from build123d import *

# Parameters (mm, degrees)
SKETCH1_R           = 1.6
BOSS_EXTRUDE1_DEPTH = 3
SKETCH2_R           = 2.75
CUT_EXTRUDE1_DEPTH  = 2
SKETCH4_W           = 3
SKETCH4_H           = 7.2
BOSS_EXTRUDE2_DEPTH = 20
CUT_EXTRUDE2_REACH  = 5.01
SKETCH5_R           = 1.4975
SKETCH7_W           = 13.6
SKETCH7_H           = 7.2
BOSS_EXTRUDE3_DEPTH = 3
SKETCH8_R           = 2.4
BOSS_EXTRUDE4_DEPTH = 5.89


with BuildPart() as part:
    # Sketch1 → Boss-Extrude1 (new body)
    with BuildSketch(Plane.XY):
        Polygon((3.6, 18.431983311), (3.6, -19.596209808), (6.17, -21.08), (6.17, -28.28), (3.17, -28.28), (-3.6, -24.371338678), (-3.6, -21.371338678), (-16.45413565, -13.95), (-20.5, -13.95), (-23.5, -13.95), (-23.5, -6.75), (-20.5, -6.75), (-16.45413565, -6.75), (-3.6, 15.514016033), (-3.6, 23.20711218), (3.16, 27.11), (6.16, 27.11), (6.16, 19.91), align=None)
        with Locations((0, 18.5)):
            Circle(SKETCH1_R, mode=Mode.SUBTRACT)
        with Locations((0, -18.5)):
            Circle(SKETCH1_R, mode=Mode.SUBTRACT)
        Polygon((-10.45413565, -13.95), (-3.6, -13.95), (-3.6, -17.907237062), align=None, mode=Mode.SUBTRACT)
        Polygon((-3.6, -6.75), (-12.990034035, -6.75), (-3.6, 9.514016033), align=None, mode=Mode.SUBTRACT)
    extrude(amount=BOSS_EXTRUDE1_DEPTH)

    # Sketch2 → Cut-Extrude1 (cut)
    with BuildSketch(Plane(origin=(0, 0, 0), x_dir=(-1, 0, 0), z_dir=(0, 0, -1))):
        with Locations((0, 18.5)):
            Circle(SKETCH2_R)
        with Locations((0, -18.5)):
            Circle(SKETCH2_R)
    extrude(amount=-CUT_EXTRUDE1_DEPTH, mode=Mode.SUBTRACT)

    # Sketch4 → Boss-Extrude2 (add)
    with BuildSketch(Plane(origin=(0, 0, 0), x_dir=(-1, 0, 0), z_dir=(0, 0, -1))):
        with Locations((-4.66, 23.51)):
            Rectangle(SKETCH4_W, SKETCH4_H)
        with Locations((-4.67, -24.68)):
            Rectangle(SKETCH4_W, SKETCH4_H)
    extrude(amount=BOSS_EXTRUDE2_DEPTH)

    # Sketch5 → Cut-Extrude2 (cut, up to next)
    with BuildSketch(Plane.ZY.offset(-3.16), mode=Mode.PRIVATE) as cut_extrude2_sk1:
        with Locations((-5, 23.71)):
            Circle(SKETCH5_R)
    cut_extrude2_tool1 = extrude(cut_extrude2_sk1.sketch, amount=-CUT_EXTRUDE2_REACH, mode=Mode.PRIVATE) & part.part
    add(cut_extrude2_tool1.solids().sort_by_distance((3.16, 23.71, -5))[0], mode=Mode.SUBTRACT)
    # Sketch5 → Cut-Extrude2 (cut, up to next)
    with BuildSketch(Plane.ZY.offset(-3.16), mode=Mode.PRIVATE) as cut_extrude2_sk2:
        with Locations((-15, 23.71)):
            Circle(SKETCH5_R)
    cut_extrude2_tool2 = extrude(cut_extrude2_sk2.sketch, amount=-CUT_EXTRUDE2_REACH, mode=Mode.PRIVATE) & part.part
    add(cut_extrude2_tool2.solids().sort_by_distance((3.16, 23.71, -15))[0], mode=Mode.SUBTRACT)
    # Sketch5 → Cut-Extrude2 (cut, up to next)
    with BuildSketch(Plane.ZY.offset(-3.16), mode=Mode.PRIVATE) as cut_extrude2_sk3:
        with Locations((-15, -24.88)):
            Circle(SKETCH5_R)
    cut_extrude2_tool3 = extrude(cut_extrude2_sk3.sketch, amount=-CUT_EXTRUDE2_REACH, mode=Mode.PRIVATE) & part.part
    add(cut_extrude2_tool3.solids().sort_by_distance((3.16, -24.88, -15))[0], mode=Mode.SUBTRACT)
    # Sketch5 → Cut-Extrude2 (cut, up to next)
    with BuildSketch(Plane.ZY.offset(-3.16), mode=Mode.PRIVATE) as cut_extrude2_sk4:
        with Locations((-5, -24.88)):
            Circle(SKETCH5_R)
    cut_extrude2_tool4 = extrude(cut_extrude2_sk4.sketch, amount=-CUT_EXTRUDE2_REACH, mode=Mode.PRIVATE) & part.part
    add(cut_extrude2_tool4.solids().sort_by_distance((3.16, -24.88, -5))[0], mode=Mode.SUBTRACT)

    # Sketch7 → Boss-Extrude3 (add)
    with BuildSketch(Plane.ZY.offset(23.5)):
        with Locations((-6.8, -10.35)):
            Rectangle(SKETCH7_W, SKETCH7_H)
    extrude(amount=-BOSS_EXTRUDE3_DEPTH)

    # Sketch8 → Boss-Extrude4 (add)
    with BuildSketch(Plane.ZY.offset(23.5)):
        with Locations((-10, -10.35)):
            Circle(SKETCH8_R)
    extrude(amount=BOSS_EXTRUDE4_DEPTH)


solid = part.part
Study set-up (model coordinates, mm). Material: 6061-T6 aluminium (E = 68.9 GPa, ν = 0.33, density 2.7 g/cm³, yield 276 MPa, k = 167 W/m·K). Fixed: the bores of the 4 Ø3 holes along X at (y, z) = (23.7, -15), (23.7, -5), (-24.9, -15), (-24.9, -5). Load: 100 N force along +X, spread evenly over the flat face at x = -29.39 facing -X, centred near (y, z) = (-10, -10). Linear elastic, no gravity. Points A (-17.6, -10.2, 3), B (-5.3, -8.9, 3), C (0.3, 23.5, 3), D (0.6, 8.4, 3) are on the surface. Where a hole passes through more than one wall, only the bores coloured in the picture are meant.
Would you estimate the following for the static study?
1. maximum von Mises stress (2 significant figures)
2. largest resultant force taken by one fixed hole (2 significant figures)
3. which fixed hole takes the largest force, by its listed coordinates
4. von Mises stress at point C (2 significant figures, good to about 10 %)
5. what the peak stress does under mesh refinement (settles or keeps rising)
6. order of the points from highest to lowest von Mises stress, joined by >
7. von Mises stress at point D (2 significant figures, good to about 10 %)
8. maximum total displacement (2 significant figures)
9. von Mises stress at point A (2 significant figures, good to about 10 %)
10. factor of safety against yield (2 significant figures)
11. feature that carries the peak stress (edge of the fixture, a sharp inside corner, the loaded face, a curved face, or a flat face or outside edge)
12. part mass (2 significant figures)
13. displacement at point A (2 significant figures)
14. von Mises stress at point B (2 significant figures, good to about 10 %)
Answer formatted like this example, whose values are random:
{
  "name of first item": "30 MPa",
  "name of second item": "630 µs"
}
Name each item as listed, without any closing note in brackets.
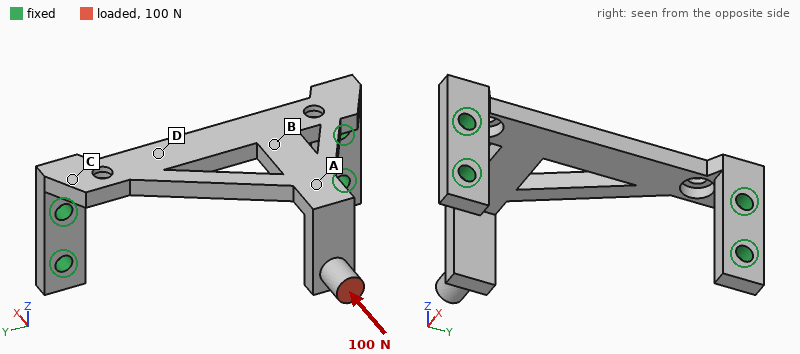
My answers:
{
  "maximum von Mises stress": "210 MPa",
  "largest resultant force taken by one fixed hole": "76 N",
  "which fixed hole takes the largest force, by its listed coordinates": "(-24.9, -5)",
  "von Mises stress at point C": "39 MPa",
  "what the peak stress does under mesh refinement": "settles",
  "order of the points from highest to lowest von Mises stress, joined by >": "A > B > C > D",
  "von Mises stress at point D": "24 MPa",
  "maximum total displacement": "0.75 mm",
  "von Mises stress at point A": "96 MPa",
  "factor of safety against yield": "1.3",
  "feature that carries the peak stress": "a curved face",
  "part mass": "8.2 g",
  "displacement at point A": "0.29 mm",
  "von Mises stress at point B": "54 MPa"
}
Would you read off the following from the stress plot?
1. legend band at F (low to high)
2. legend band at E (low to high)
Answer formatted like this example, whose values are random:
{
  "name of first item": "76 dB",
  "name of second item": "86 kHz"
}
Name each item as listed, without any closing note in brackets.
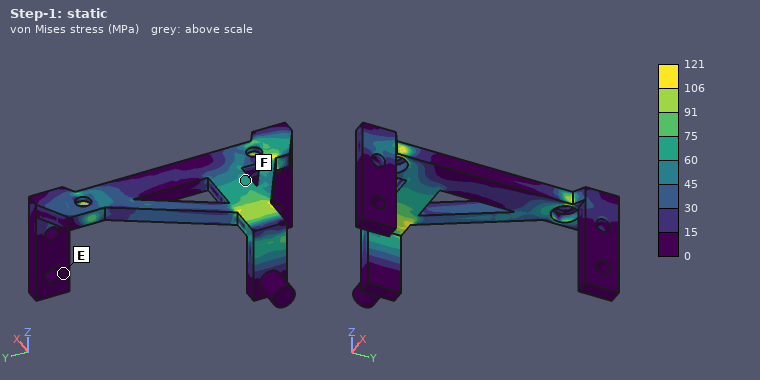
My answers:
{
  "legend band at F": "60 to 75 MPa",
  "legend band at E": "0 to 15 MPa"
}
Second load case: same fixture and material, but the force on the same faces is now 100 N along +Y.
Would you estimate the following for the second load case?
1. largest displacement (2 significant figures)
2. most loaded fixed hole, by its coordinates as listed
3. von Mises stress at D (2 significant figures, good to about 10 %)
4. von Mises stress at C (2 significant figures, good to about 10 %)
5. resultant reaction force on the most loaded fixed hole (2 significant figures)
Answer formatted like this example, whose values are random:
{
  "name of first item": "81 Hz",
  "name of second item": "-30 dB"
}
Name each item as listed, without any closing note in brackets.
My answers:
{
  "largest displacement": "0.27 mm",
  "most loaded fixed hole, by its coordinates as listed": "(23.7, -5)",
  "von Mises stress at D": "19 MPa",
  "von Mises stress at C": "17 MPa",
  "resultant reaction force on the most loaded fixed hole": "120 N"
}
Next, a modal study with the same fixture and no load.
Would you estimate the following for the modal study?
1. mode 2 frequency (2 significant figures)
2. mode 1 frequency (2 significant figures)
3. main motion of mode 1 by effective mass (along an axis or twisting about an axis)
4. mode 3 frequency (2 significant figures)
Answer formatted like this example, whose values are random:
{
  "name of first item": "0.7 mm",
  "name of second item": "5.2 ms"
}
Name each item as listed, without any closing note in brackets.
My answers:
{
  "mode 2 frequency": "3700 Hz",
  "mode 1 frequency": "1200 Hz",
  "main motion of mode 1 by effective mass": "along Z",
  "mode 3 frequency": "4400 Hz"
}
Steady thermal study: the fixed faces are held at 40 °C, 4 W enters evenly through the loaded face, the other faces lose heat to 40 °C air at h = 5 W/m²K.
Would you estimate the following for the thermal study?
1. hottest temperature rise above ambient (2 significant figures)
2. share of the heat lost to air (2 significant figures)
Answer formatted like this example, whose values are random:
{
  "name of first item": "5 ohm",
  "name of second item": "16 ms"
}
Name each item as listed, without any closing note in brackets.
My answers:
{
  "hottest temperature rise above ambient": "47 K",
  "share of the heat lost to air": "4.6 %"
}
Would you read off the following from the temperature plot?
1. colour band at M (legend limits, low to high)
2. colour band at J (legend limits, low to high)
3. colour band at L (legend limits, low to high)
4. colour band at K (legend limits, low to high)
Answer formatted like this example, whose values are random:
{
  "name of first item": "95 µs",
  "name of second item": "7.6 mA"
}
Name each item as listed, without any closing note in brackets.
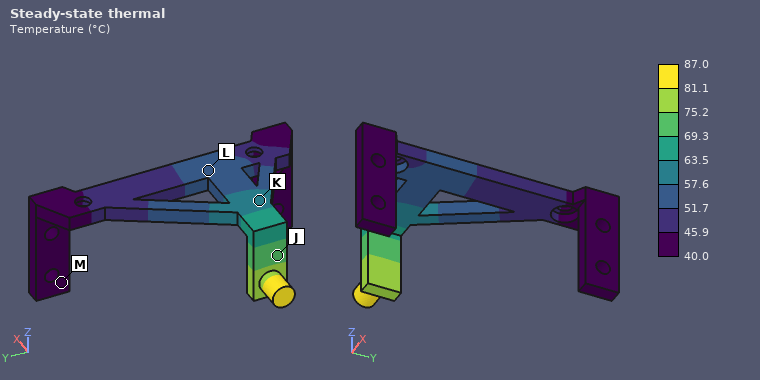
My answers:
{
  "colour band at M": "40.0 to 45.9 °C",
  "colour band at J": "69.3 to 75.2 °C",
  "colour band at L": "51.7 to 57.6 °C",
  "colour band at K": "57.6 to 63.5 °C"
}
